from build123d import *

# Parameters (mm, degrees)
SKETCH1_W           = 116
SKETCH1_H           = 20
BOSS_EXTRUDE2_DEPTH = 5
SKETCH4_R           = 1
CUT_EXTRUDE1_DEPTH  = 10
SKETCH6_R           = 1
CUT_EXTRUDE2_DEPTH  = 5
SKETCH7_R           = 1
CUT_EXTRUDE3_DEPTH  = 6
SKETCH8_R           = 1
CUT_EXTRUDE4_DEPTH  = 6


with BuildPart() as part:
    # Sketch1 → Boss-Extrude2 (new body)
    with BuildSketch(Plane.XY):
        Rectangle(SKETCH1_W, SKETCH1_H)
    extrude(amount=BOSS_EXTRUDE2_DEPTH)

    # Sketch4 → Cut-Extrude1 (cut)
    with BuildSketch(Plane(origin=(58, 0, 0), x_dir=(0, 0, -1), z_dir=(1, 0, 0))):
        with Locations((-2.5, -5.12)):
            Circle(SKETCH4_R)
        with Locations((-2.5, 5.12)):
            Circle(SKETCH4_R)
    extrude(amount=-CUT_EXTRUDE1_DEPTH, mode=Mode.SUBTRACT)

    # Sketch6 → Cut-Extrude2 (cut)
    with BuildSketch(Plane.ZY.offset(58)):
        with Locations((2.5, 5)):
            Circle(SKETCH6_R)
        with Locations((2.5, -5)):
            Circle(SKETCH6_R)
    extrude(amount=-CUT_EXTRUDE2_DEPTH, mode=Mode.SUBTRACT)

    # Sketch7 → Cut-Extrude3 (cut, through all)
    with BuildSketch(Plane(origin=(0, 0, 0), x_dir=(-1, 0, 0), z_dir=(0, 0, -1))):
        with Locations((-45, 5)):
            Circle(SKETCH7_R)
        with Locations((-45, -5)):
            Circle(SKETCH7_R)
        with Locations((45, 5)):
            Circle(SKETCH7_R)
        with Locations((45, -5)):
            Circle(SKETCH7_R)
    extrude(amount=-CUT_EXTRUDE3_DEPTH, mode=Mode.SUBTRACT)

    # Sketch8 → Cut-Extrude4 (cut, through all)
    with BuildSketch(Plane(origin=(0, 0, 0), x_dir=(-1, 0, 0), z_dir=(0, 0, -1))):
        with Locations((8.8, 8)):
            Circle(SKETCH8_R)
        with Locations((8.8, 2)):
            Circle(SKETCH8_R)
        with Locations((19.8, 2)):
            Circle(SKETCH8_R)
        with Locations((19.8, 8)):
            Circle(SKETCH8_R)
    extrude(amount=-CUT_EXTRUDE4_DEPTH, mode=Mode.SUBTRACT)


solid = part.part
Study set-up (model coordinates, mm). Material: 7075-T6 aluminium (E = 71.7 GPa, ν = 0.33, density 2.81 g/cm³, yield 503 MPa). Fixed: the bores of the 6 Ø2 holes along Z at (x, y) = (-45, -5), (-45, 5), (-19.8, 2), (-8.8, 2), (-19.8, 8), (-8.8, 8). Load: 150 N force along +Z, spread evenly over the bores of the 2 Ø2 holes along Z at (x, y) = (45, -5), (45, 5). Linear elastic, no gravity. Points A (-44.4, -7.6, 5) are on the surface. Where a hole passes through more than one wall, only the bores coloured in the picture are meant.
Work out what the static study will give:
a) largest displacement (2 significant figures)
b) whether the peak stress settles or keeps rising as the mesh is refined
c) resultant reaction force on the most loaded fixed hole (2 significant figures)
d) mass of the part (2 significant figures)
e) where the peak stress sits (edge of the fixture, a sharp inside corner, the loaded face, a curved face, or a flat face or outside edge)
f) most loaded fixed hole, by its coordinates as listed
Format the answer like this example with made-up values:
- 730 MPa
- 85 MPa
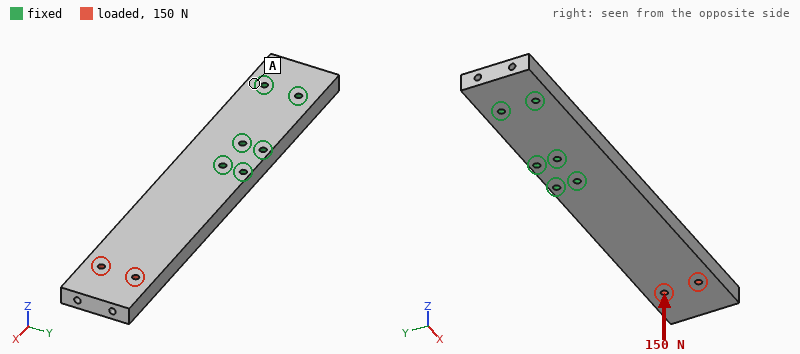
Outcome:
- 0.75 mm
- keeps rising
- 410 N
- 32 g
- edge of the fixture
- (-8.8, 2)
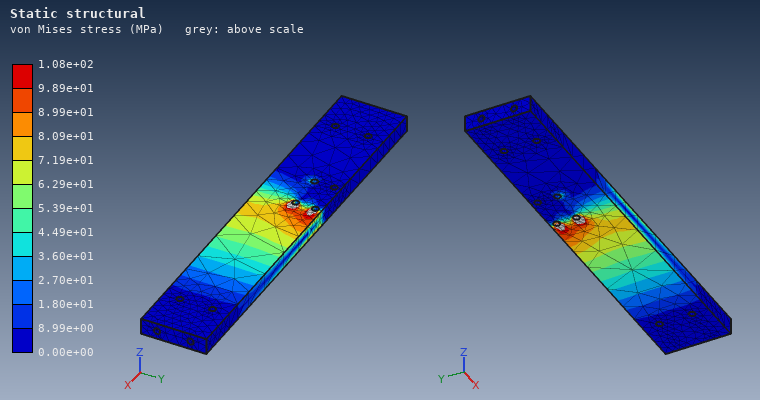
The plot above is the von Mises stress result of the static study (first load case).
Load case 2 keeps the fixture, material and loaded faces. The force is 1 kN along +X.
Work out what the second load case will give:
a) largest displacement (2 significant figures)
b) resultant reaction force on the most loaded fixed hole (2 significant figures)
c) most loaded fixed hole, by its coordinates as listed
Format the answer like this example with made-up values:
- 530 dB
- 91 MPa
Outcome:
- 13 µm
- 560 N
- (-8.8, 2)
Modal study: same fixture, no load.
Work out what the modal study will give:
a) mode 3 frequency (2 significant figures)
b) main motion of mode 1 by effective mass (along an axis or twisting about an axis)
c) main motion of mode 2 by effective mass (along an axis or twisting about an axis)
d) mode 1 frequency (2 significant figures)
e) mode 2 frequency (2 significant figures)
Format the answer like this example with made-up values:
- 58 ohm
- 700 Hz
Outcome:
- 5100 Hz
- along Z
- along Y
- 910 Hz
- 3100 Hz
